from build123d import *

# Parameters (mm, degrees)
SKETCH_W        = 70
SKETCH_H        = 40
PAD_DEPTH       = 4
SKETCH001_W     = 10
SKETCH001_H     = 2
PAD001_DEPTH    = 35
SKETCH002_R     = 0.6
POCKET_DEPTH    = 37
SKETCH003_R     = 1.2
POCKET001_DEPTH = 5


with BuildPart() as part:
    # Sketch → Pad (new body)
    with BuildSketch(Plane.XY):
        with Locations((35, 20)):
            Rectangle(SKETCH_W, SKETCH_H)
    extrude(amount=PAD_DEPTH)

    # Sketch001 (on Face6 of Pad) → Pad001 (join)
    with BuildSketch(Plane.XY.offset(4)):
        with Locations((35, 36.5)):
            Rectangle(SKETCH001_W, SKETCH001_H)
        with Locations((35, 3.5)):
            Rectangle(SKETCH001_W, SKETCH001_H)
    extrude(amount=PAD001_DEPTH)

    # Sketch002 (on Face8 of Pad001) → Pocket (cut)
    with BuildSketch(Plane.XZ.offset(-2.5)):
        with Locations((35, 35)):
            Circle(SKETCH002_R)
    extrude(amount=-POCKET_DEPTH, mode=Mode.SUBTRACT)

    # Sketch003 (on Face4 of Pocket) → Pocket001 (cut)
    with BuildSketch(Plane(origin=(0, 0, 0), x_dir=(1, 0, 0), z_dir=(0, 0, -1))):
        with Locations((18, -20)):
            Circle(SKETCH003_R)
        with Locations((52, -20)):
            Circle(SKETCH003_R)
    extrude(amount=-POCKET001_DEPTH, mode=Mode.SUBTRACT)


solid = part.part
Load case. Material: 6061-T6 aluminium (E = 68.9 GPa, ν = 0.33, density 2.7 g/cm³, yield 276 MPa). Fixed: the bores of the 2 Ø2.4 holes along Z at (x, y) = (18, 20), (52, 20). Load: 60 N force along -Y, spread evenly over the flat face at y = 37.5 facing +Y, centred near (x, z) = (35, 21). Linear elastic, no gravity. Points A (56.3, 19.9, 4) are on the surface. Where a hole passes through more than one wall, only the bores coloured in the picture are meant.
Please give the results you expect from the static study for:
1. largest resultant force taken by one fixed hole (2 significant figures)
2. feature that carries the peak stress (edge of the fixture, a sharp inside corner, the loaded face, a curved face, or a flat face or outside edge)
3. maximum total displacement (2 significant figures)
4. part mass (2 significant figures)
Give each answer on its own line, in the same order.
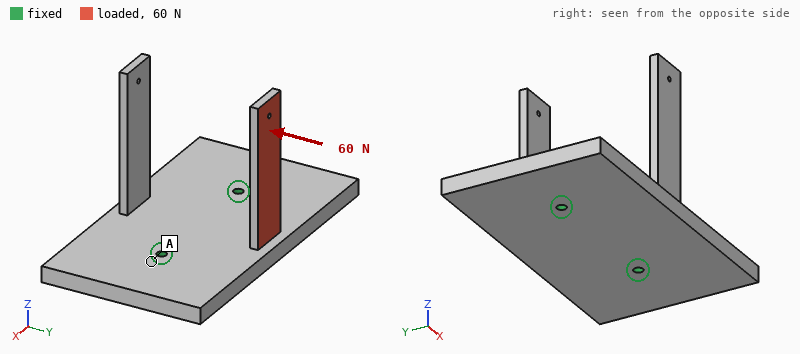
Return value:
31 N
the loaded face
0.78 mm
34 g
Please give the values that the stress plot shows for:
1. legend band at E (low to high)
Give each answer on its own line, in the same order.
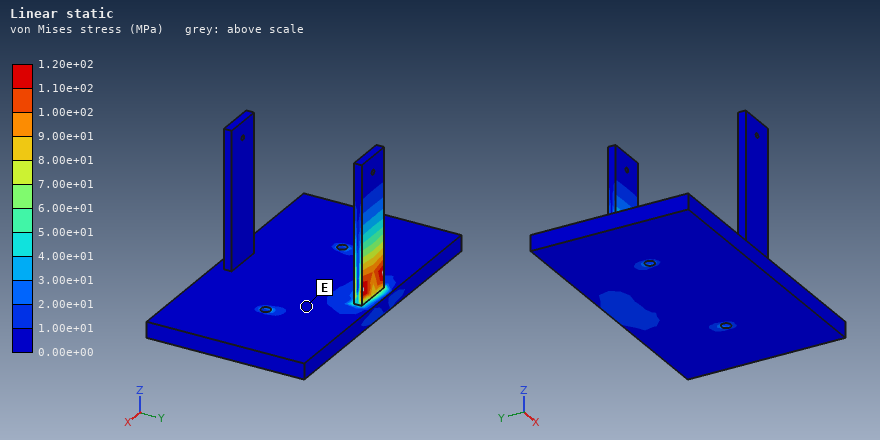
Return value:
0.00e+00 to 1.00e+01 MPa
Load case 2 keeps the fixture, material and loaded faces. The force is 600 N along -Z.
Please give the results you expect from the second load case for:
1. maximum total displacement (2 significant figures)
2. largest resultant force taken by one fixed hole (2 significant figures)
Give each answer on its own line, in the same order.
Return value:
0.84 mm
300 N
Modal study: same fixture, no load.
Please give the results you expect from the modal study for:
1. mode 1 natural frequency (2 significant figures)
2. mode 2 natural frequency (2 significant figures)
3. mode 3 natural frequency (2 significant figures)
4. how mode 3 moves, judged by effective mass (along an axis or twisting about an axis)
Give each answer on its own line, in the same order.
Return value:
1300 Hz
1300 Hz
4100 Hz
twisting about X
